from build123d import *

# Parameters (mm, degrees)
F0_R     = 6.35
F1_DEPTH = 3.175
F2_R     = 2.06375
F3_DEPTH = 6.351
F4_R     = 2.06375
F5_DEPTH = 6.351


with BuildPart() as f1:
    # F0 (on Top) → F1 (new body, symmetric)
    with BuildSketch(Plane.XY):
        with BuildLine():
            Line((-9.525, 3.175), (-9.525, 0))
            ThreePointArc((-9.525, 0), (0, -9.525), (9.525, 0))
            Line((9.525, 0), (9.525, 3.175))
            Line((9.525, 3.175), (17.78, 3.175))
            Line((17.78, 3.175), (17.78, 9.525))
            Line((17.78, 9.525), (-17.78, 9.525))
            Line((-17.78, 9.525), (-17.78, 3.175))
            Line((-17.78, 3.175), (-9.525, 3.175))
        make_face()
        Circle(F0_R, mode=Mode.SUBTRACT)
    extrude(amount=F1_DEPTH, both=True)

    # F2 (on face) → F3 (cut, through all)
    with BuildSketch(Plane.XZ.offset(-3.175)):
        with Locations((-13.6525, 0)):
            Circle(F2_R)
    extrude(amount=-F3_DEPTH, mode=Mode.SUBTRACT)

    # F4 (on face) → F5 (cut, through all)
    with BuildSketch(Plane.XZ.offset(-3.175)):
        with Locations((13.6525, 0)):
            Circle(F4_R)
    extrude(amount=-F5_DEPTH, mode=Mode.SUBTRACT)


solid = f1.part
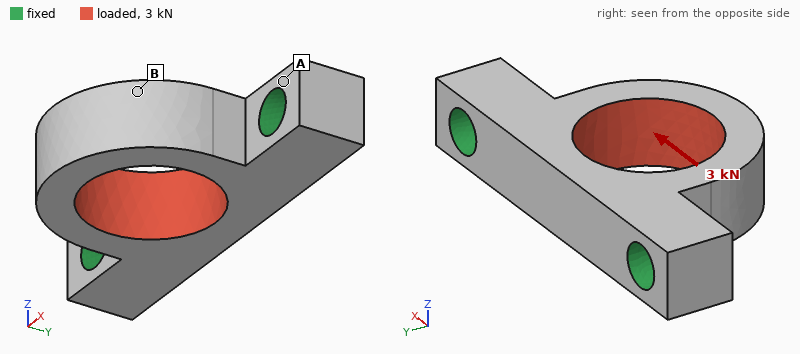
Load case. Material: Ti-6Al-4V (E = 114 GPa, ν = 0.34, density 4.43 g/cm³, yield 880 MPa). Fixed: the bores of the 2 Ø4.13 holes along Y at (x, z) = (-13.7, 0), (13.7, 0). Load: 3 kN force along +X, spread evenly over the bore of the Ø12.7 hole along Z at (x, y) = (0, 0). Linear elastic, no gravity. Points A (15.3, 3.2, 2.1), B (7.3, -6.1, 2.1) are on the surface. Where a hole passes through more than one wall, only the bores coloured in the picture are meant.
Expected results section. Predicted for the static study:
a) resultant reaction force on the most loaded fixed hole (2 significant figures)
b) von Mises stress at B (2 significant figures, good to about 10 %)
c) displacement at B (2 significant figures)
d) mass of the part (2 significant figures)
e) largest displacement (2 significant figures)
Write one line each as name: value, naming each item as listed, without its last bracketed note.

resultant reaction force on the most loaded fixed hole: 1.6 kN
von Mises stress at B: 110 MPa
displacement at B: 40 µm
mass of the part: 7.7 g
largest displacement: 42 µm
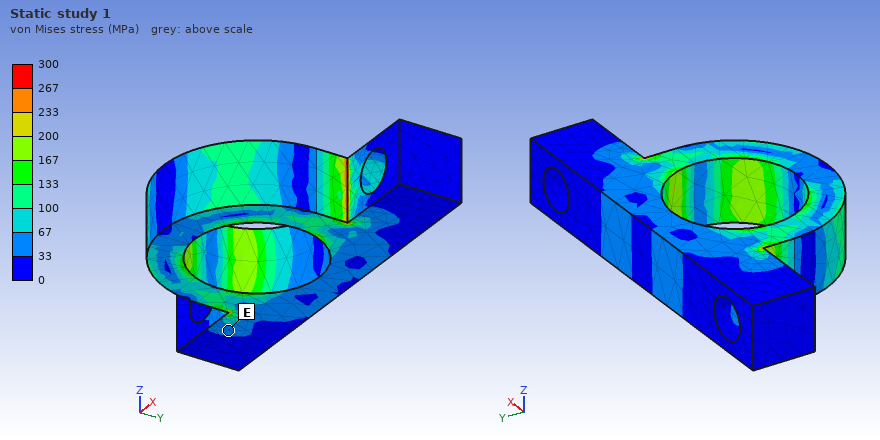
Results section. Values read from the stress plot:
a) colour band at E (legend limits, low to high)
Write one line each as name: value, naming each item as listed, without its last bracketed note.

colour band at E: 33 to 67 MPa
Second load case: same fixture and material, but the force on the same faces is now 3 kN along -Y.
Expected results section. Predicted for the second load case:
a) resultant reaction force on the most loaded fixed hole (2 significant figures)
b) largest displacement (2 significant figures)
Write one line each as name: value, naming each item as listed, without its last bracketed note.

resultant reaction force on the most loaded fixed hole: 1.5 kN
largest displacement: 13 µm
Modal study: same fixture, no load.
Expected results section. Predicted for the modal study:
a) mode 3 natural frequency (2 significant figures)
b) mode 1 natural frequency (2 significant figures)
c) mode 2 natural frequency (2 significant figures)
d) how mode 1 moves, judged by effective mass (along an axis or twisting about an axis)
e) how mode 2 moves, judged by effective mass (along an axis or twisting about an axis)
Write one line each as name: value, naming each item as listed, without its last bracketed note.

mode 3 natural frequency: 31 kHz
mode 1 natural frequency: 13 kHz
mode 2 natural frequency: 22 kHz
how mode 1 moves, judged by effective mass: along Z
how mode 2 moves, judged by effective mass: along X
